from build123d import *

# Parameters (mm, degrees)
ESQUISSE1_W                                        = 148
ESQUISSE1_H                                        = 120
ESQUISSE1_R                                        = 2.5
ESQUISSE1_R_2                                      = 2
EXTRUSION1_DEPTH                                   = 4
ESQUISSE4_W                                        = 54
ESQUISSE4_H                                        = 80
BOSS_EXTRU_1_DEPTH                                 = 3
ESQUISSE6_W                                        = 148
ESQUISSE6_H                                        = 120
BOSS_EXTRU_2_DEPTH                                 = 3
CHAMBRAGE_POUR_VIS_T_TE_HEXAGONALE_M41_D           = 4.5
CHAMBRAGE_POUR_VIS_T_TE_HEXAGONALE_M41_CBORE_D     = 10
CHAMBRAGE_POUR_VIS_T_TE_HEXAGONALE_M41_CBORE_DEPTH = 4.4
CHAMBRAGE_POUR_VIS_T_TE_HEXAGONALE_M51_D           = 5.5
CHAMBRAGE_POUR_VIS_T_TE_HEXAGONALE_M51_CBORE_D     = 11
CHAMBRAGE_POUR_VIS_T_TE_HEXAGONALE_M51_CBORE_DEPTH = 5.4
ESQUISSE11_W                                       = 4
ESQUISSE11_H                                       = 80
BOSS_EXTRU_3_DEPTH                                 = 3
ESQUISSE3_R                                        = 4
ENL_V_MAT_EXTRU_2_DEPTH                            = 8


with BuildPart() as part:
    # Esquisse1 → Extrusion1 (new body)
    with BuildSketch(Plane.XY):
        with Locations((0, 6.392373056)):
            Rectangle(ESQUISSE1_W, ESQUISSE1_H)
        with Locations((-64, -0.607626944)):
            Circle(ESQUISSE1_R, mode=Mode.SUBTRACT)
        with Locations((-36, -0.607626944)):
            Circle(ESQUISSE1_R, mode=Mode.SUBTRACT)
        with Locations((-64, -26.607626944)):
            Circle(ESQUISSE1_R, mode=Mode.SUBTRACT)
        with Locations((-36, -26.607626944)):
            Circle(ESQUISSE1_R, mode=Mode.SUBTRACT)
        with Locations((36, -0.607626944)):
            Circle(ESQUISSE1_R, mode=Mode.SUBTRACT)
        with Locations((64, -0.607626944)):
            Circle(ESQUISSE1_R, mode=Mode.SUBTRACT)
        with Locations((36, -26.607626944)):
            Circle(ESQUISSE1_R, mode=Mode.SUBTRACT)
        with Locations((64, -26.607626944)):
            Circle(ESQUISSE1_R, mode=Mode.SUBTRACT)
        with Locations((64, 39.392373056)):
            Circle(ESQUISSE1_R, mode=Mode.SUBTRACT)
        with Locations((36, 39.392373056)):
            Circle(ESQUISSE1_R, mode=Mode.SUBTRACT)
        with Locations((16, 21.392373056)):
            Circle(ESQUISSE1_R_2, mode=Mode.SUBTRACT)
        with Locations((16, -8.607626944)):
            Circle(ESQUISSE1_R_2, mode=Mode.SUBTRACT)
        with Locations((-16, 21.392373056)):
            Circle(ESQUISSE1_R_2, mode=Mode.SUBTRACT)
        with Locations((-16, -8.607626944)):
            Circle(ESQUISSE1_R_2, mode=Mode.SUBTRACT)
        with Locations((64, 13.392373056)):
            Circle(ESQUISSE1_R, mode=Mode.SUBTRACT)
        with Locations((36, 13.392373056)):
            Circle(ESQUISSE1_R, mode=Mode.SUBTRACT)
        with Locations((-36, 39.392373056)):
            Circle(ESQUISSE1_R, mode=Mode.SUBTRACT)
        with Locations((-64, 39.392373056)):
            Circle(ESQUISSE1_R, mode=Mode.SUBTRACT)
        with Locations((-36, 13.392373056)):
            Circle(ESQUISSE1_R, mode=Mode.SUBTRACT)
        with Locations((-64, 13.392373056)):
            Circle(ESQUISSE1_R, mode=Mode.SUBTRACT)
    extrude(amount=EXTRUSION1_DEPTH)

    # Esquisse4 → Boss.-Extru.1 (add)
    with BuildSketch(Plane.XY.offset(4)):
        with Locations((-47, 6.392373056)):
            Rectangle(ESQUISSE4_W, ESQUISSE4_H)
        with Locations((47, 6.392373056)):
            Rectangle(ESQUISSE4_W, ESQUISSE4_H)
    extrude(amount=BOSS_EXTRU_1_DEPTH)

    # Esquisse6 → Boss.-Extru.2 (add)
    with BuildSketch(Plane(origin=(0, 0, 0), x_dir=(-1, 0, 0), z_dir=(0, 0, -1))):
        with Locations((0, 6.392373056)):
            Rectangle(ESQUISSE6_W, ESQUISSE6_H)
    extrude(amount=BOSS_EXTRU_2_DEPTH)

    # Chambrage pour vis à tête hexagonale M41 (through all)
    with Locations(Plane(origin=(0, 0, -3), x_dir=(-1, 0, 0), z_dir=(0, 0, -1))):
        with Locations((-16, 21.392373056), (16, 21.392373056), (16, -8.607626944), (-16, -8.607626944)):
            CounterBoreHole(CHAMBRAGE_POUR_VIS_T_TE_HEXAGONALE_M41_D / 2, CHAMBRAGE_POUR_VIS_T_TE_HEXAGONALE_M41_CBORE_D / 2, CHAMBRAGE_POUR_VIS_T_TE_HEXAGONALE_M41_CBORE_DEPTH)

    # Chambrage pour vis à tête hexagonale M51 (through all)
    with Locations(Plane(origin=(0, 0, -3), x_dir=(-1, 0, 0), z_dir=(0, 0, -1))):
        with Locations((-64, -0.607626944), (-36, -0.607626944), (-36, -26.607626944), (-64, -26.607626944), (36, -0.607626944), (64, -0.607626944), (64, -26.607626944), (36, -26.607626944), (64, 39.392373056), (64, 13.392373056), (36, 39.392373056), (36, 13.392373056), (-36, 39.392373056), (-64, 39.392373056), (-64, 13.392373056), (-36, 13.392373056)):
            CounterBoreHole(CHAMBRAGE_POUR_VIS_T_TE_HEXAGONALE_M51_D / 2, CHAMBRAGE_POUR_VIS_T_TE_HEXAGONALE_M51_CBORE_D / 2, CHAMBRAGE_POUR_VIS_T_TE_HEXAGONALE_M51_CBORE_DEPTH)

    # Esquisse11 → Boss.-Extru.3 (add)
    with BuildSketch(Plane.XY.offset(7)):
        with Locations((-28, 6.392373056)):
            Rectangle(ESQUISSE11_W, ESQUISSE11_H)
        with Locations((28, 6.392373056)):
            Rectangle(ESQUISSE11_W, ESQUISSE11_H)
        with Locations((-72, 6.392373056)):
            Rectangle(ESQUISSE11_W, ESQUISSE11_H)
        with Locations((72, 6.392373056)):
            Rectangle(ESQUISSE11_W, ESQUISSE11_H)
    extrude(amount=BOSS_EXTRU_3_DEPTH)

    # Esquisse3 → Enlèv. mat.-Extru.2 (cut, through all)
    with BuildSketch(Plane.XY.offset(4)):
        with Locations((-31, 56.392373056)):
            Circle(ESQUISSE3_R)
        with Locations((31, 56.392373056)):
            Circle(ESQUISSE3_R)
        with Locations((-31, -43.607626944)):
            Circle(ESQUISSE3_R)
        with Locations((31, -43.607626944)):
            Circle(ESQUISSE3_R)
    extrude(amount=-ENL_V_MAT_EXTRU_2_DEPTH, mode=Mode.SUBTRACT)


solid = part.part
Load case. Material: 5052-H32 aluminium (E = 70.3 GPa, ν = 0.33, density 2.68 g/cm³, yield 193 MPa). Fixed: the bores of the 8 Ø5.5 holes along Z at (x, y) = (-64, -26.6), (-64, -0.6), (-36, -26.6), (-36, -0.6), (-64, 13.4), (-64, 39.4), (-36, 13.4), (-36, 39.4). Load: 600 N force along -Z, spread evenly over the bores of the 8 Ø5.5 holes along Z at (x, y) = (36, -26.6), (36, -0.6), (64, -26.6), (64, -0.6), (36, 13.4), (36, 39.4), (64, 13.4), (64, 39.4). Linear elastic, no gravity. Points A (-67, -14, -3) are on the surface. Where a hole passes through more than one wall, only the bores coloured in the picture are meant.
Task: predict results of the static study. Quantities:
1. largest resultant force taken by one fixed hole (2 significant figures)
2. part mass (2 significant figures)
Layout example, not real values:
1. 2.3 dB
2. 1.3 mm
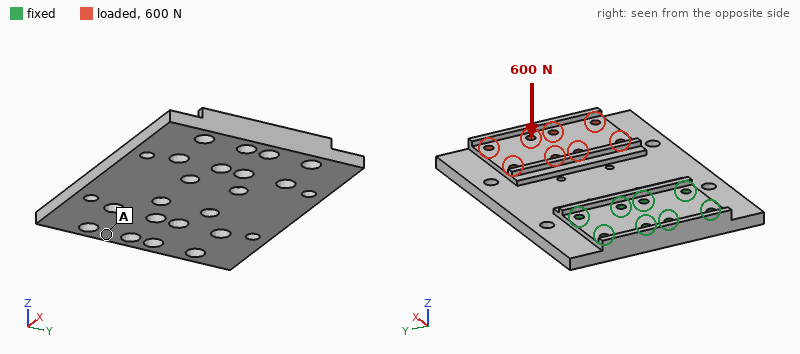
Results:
1. 870 N
2. 380 g
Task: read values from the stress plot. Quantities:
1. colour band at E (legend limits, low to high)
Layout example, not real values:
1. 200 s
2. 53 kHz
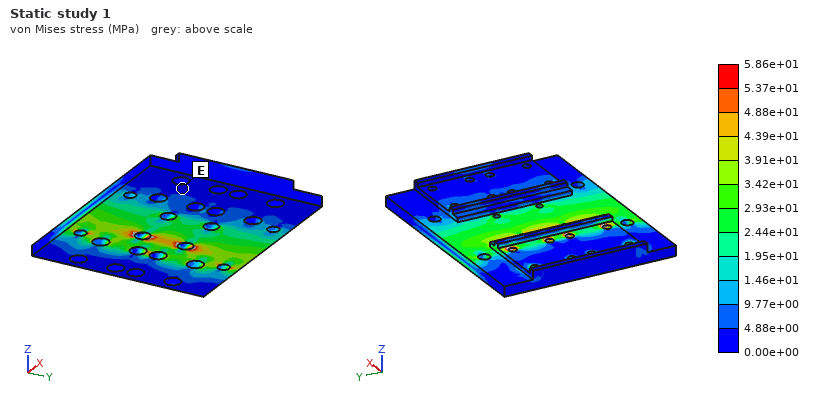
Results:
1. 0.00e+00 to 4.88e+00 MPa
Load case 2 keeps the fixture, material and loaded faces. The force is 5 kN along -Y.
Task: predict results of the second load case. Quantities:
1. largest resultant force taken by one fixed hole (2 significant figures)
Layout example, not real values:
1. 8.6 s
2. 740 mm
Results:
1. 4.0 kN
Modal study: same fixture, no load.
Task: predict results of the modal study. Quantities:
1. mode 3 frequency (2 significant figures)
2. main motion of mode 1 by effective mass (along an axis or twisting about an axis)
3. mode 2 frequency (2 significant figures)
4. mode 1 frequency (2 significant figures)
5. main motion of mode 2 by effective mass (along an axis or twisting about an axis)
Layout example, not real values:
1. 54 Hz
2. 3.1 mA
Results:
1. 2900 Hz
2. along Z
3. 1100 Hz
4. 470 Hz
5. twisting about X
